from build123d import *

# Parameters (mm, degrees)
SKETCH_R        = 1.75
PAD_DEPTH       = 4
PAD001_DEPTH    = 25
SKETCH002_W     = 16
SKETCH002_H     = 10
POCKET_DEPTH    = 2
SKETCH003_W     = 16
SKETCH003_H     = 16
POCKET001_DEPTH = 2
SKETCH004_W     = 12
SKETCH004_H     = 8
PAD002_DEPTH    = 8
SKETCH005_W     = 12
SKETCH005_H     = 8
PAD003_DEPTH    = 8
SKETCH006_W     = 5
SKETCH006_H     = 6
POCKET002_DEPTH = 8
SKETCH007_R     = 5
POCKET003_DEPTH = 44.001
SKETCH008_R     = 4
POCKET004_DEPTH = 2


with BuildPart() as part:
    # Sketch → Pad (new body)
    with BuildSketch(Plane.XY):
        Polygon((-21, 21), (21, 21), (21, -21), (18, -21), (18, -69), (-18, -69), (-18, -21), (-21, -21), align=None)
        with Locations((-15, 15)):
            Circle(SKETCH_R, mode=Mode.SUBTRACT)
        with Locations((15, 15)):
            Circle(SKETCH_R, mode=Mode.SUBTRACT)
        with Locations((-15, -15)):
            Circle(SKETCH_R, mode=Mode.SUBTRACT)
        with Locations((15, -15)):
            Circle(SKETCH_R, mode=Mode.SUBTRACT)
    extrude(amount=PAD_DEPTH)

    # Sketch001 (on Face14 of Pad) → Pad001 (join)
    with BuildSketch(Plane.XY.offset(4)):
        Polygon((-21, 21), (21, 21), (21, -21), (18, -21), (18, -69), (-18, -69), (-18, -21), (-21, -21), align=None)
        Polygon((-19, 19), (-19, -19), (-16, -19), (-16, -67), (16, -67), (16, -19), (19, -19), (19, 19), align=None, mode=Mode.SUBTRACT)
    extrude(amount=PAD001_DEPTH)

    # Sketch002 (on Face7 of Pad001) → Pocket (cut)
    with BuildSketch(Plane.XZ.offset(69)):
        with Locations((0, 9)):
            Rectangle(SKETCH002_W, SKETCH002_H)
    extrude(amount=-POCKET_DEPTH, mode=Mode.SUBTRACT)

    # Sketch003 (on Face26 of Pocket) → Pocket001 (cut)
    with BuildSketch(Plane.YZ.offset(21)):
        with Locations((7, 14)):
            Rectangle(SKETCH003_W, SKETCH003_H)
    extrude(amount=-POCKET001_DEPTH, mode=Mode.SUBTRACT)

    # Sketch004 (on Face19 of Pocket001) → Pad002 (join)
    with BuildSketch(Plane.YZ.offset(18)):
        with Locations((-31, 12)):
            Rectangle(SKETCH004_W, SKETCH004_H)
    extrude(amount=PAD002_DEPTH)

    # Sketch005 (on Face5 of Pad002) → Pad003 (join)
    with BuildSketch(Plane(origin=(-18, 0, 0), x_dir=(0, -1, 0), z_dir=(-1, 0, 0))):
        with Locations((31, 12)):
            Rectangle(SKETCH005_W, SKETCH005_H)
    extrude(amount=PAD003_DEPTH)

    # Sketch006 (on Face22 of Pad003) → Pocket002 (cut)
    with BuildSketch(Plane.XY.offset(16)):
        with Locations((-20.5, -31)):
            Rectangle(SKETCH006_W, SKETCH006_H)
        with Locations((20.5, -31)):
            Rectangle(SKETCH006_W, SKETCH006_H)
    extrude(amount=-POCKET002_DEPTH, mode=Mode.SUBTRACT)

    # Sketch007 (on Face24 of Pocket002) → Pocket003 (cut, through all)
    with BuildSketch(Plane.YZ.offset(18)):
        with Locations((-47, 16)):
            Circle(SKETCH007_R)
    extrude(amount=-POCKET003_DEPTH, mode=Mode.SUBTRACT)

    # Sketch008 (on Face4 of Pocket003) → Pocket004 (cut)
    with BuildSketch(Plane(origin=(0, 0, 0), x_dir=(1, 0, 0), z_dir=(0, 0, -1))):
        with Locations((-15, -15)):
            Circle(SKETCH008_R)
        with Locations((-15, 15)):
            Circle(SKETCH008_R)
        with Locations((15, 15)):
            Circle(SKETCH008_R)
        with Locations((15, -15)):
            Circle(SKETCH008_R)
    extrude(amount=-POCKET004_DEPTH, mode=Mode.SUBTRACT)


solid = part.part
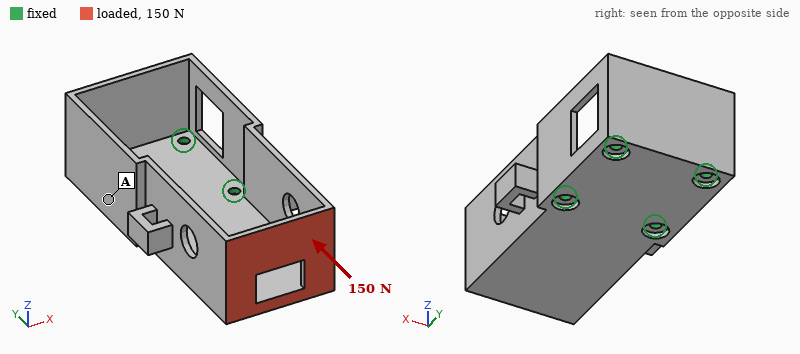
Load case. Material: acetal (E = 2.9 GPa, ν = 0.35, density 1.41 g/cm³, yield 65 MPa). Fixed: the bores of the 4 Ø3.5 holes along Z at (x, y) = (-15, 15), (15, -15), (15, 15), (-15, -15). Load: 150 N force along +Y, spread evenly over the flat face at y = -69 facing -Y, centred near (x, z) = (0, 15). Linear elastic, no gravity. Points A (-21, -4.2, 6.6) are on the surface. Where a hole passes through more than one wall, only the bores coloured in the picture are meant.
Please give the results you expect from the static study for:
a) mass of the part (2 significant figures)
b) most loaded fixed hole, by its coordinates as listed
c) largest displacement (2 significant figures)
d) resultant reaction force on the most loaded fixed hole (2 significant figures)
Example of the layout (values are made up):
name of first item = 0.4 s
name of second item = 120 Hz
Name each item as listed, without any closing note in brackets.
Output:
mass of the part = 37 g
most loaded fixed hole, by its coordinates as listed = (15, -15)
largest displacement = 0.75 mm
resultant reaction force on the most loaded fixed hole = 67 N
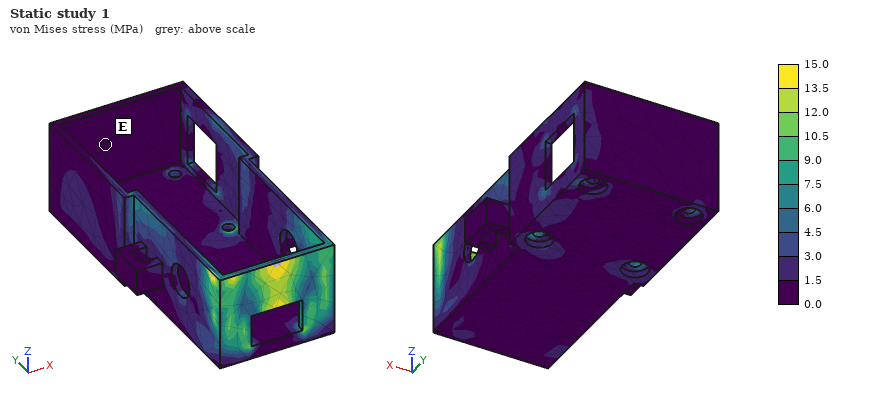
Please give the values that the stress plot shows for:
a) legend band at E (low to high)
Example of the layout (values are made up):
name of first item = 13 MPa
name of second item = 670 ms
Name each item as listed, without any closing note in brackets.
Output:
legend band at E = 0.0 to 1.5 MPa
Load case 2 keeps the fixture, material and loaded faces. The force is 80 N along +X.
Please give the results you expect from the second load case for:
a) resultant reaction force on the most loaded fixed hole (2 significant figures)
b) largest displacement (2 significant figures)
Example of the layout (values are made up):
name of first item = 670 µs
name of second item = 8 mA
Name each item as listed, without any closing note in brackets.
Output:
resultant reaction force on the most loaded fixed hole = 150 N
largest displacement = 1.0 mm
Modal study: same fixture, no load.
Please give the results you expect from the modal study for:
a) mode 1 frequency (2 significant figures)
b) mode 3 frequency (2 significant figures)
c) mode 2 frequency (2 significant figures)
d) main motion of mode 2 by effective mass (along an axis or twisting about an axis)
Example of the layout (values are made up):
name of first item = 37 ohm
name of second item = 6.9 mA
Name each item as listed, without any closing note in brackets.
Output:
mode 1 frequency = 550 Hz
mode 3 frequency = 930 Hz
mode 2 frequency = 620 Hz
main motion of mode 2 by effective mass = along Z
